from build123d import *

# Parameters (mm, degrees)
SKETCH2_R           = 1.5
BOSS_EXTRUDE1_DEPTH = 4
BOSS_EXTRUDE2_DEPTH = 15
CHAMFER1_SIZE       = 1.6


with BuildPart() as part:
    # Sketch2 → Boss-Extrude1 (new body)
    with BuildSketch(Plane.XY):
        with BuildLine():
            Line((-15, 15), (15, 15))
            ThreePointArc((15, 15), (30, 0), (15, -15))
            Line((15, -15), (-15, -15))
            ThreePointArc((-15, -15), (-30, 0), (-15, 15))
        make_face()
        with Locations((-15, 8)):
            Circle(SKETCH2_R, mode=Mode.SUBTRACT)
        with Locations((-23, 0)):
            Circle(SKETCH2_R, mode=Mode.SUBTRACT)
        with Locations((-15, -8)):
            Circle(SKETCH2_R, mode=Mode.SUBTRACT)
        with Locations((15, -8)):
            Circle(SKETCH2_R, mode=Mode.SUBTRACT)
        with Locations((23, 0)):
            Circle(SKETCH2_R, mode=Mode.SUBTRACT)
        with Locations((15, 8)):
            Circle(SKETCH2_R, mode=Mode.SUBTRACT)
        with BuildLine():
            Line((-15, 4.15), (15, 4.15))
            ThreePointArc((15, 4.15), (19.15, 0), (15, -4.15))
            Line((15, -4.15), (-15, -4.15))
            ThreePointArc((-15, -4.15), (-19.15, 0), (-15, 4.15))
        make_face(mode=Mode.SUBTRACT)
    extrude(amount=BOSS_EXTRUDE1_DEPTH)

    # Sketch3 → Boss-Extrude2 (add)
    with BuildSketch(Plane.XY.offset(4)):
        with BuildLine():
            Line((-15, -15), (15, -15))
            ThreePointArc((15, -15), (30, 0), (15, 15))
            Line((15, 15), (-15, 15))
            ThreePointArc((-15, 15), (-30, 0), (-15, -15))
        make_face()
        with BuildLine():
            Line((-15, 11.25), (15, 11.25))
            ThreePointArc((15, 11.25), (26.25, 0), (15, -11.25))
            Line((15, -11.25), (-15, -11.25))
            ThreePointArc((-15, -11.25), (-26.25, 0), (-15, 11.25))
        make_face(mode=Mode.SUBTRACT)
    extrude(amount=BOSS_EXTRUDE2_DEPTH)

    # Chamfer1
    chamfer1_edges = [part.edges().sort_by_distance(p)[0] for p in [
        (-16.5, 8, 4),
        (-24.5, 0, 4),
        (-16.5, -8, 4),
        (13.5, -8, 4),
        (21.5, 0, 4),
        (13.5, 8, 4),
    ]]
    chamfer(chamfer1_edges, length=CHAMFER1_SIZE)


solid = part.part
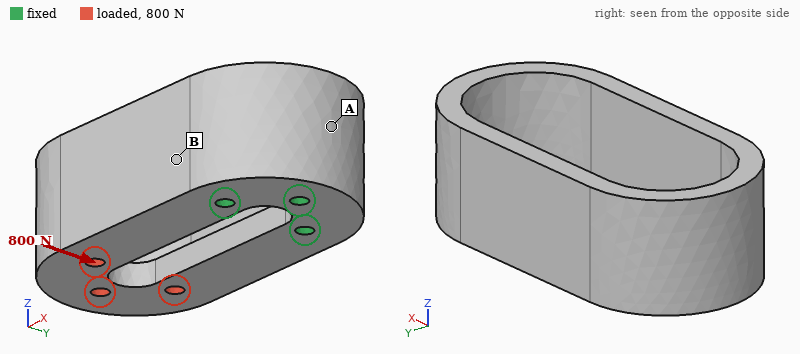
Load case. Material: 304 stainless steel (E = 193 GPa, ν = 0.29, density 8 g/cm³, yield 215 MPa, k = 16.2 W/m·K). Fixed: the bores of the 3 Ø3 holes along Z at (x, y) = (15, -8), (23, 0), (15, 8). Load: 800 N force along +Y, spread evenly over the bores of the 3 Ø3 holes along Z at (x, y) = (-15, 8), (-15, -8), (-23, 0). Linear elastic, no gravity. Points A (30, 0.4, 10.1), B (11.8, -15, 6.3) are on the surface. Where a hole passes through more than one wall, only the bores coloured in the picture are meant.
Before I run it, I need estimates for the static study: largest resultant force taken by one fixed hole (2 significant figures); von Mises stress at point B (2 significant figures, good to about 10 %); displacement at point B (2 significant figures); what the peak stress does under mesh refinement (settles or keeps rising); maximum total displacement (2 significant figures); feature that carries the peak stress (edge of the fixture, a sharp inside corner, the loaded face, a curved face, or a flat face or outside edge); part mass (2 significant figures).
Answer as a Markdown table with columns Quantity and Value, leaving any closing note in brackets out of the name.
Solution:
| Quantity | Value |
|---|---|
| largest resultant force taken by one fixed hole | 1.2 kN |
| von Mises stress at point B | 37 MPa |
| displacement at point B | 7.2 µm |
| what the peak stress does under mesh refinement | keeps rising |
| maximum total displacement | 41 µm |
| feature that carries the peak stress | edge of the fixture |
| part mass | 100 g |
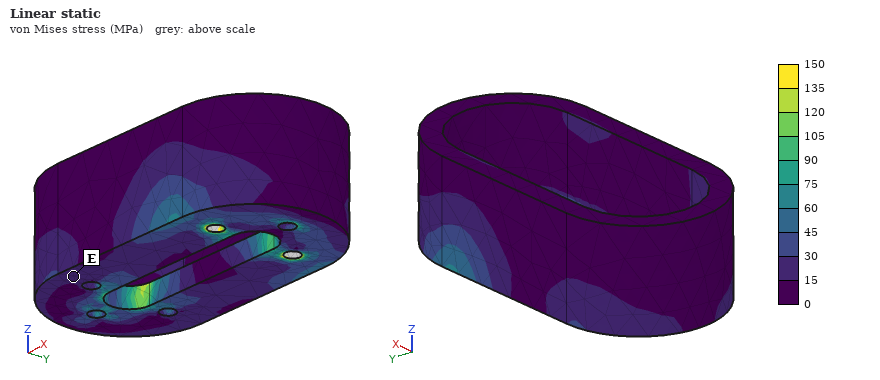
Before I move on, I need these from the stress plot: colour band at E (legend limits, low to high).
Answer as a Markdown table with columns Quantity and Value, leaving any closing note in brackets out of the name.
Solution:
| Quantity | Value |
|---|---|
| colour band at E | 15 to 30 MPa |
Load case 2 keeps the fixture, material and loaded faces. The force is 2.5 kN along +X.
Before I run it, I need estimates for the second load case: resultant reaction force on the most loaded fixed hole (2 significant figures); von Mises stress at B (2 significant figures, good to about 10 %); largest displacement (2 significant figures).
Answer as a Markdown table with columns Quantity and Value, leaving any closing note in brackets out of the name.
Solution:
| Quantity | Value |
|---|---|
| resultant reaction force on the most loaded fixed hole | 1.2 kN |
| von Mises stress at B | 10 MPa |
| largest displacement | 14 µm |
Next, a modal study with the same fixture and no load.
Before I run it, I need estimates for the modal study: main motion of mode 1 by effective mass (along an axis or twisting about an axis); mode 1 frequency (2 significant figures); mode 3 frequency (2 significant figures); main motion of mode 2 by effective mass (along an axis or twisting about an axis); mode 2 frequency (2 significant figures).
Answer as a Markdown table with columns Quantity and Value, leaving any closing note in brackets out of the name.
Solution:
| Quantity | Value |
|---|---|
| main motion of mode 1 by effective mass | along Z |
| mode 1 frequency | 2500 Hz |
| mode 3 frequency | 5800 Hz |
| main motion of mode 2 by effective mass | along Y |
| mode 2 frequency | 3000 Hz |
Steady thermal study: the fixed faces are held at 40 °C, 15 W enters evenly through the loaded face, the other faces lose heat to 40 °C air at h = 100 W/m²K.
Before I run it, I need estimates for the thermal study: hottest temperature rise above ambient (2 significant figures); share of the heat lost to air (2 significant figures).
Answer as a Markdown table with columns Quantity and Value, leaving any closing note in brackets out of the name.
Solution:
| Quantity | Value |
|---|---|
| hottest temperature rise above ambient | 76 K |
| share of the heat lost to air | 90 % |
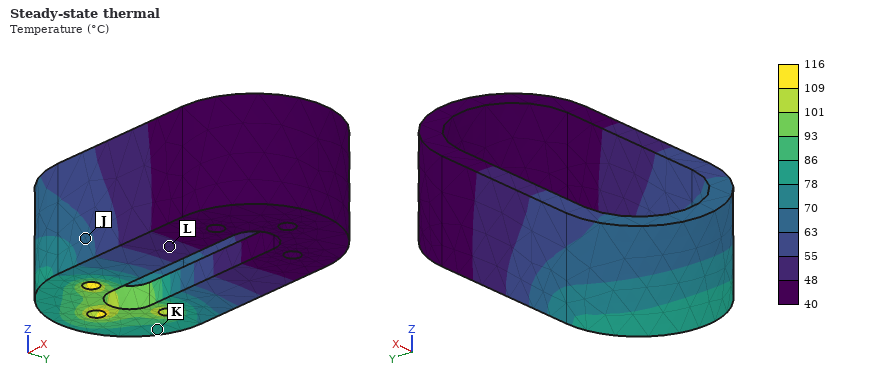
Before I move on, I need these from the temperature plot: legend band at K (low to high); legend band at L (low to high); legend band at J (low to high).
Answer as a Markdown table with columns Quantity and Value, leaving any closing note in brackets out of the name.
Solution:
| Quantity | Value |
|---|---|
| legend band at K | 78 to 86 °C |
| legend band at L | 48 to 55 °C |
| legend band at J | 63 to 70 °C |
